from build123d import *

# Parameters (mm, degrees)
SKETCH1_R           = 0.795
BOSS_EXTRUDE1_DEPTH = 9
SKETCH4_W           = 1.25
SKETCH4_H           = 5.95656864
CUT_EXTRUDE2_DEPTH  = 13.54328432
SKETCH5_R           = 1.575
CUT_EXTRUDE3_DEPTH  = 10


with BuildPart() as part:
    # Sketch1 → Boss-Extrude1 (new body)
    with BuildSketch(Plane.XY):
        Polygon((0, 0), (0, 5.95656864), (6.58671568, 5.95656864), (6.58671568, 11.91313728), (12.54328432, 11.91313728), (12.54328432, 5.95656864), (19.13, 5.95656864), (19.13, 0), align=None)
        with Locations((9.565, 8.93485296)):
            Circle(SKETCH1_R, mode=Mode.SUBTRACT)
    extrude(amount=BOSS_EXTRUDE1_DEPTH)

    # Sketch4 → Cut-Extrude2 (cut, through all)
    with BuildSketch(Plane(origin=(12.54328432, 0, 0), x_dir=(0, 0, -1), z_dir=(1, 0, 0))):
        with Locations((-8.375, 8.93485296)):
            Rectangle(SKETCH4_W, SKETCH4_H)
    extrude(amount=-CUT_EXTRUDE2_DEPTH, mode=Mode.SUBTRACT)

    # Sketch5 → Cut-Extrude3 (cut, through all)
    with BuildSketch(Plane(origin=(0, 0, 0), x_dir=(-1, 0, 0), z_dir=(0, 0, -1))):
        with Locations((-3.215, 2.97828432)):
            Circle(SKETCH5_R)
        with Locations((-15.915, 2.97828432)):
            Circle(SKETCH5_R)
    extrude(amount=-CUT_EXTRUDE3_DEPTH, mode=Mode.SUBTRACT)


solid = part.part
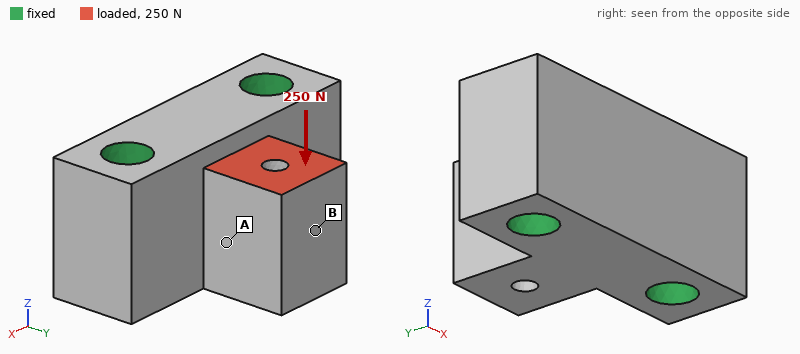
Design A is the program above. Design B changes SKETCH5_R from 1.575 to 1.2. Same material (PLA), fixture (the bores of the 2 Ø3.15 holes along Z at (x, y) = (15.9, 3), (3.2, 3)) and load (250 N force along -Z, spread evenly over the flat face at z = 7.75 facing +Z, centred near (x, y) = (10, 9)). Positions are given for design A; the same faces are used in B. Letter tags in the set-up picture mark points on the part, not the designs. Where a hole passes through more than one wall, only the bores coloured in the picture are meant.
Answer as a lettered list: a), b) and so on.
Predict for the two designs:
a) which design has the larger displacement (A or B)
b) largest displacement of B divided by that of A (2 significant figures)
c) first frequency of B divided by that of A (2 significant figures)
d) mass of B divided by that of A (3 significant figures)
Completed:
a) B
b) 1.1
c) 0.95
d) 1.05
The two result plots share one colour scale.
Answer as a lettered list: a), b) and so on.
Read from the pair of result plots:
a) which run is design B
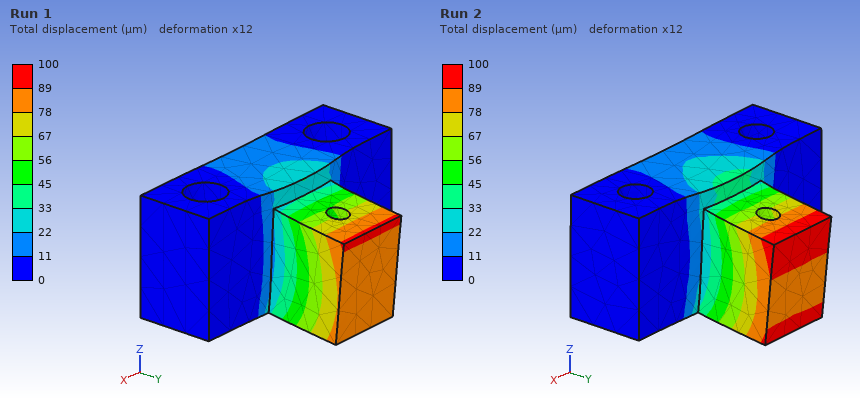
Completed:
a) Run 2
